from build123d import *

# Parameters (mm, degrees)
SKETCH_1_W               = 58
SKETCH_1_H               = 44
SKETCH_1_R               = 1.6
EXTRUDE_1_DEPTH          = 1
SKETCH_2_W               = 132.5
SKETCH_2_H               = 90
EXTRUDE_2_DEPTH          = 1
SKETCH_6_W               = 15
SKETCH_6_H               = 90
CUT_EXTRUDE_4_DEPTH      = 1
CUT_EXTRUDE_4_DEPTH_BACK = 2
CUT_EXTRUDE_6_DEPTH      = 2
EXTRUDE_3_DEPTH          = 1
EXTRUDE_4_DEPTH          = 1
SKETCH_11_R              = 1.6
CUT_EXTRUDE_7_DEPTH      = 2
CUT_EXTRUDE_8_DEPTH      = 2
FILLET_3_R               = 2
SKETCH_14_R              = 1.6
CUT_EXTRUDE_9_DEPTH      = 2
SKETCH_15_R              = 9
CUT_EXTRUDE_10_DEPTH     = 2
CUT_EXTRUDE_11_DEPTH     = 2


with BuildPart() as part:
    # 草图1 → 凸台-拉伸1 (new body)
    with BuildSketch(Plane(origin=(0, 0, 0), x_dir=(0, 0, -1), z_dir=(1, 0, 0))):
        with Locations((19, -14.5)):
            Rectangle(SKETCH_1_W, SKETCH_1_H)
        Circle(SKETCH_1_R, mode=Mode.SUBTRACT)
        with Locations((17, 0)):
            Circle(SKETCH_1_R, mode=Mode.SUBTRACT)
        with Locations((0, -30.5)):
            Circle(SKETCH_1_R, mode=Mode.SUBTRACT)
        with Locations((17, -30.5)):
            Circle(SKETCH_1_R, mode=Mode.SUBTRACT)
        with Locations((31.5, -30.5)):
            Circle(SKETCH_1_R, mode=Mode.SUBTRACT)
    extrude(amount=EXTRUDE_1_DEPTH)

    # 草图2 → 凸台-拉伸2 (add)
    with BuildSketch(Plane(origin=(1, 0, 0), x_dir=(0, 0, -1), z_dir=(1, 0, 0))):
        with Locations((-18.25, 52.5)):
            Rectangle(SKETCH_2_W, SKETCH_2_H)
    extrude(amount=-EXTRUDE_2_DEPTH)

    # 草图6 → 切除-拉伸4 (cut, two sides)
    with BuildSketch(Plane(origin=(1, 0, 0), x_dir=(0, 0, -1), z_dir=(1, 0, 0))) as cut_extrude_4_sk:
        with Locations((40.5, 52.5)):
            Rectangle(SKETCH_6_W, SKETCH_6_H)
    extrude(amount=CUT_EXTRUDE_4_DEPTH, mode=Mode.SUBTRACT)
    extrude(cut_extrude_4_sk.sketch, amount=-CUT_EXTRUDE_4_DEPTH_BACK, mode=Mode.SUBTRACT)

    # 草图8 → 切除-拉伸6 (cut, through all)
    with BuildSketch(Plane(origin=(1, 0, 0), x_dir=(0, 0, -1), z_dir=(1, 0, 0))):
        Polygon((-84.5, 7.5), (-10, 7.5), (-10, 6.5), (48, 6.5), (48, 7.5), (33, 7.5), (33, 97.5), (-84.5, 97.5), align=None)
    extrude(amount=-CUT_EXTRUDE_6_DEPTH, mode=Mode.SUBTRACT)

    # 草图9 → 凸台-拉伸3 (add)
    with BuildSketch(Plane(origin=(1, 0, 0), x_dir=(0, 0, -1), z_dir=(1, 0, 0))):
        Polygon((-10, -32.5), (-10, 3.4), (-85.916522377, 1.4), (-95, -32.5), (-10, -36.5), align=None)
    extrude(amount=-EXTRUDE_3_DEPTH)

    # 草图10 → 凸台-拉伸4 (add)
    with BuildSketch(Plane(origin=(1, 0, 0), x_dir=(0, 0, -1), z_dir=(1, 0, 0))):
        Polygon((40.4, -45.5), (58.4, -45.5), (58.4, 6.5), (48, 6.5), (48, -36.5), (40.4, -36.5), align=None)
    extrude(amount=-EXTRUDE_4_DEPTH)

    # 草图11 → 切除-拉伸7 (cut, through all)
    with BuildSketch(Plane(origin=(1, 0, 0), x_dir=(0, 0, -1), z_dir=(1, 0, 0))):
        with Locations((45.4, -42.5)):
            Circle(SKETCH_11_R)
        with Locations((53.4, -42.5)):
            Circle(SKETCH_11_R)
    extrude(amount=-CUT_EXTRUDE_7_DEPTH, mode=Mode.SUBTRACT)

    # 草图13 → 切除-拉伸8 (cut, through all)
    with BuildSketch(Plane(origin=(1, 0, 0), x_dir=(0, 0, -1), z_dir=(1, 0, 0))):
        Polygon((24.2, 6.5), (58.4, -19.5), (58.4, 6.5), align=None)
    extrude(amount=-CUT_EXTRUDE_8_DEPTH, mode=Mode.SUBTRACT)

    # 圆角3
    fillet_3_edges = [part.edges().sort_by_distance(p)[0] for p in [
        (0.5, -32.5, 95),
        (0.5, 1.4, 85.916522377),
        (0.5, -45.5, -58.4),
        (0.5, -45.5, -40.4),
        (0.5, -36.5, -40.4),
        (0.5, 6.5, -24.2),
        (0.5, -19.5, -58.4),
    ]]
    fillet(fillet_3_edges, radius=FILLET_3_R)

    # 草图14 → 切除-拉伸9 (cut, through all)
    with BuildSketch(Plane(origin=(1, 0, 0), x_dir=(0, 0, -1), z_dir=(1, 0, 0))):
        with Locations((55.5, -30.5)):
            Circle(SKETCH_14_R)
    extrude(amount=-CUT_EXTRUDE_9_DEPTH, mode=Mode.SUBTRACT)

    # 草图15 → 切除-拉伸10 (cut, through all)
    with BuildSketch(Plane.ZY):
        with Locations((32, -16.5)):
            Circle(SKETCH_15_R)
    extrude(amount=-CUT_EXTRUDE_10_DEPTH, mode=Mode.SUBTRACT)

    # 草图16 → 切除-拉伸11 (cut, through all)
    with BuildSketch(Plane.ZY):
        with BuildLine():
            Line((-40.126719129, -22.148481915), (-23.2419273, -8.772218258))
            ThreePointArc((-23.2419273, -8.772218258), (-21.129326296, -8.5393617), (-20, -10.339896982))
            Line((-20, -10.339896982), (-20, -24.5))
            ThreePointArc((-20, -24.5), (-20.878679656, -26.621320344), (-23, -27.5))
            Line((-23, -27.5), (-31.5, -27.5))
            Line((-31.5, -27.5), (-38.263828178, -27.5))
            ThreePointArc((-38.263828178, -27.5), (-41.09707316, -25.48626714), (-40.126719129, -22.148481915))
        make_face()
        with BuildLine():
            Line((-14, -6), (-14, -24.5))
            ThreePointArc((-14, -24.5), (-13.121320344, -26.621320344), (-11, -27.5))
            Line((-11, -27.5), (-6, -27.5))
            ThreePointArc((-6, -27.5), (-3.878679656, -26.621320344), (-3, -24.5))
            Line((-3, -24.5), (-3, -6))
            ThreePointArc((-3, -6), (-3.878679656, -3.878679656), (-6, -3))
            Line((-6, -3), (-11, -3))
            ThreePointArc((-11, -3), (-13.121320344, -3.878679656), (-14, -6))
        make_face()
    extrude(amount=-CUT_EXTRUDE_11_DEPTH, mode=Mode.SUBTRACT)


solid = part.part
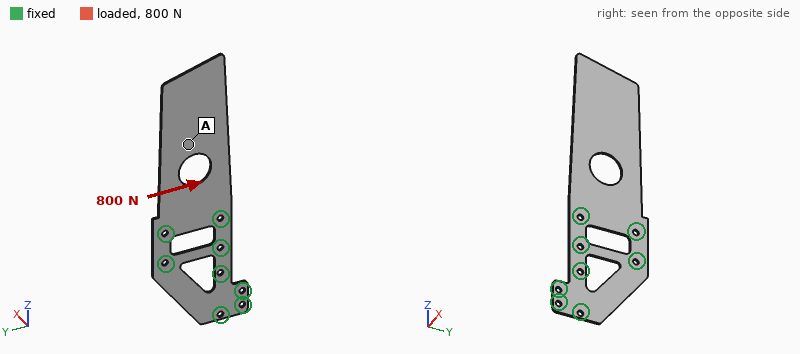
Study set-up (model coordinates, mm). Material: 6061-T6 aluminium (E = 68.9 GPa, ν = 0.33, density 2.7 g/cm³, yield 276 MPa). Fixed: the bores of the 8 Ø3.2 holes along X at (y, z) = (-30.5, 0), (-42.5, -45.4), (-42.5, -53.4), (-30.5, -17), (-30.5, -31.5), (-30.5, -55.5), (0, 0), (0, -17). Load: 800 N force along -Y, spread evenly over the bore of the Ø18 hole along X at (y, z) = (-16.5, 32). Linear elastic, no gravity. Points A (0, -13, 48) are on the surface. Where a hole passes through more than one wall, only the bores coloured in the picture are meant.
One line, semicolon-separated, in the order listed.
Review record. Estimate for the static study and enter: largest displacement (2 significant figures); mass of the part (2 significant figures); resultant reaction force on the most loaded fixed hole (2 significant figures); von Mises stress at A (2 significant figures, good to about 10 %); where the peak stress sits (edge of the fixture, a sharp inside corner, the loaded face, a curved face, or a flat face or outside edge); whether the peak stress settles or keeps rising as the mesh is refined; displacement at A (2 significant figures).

0.16 mm; 13 g; 830 N; 16 MPa; edge of the fixture; keeps rising; 0.10 mm
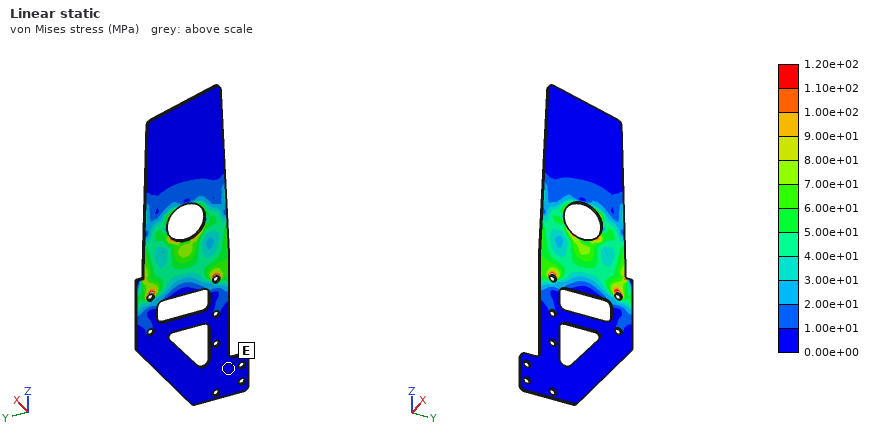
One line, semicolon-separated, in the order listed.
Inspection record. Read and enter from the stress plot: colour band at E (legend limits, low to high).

0.00e+00 to 1.00e+01 MPa
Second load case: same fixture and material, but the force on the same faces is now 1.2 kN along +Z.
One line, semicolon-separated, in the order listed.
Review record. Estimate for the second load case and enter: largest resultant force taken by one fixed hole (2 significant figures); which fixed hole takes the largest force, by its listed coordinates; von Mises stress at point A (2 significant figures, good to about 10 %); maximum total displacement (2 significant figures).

610 N; (-30.5, 0); 15 MPa; 27 µm
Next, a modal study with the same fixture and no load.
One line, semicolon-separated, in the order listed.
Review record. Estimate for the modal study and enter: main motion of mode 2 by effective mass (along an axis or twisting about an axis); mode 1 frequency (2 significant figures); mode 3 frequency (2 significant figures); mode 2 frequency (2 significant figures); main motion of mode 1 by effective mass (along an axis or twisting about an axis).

twisting about Z; 97 Hz; 630 Hz; 520 Hz; along X
